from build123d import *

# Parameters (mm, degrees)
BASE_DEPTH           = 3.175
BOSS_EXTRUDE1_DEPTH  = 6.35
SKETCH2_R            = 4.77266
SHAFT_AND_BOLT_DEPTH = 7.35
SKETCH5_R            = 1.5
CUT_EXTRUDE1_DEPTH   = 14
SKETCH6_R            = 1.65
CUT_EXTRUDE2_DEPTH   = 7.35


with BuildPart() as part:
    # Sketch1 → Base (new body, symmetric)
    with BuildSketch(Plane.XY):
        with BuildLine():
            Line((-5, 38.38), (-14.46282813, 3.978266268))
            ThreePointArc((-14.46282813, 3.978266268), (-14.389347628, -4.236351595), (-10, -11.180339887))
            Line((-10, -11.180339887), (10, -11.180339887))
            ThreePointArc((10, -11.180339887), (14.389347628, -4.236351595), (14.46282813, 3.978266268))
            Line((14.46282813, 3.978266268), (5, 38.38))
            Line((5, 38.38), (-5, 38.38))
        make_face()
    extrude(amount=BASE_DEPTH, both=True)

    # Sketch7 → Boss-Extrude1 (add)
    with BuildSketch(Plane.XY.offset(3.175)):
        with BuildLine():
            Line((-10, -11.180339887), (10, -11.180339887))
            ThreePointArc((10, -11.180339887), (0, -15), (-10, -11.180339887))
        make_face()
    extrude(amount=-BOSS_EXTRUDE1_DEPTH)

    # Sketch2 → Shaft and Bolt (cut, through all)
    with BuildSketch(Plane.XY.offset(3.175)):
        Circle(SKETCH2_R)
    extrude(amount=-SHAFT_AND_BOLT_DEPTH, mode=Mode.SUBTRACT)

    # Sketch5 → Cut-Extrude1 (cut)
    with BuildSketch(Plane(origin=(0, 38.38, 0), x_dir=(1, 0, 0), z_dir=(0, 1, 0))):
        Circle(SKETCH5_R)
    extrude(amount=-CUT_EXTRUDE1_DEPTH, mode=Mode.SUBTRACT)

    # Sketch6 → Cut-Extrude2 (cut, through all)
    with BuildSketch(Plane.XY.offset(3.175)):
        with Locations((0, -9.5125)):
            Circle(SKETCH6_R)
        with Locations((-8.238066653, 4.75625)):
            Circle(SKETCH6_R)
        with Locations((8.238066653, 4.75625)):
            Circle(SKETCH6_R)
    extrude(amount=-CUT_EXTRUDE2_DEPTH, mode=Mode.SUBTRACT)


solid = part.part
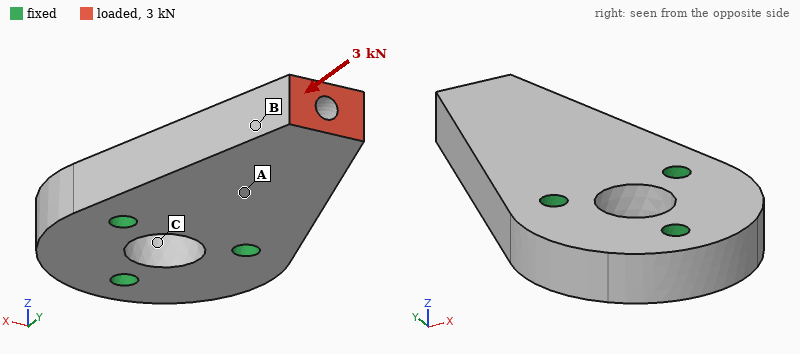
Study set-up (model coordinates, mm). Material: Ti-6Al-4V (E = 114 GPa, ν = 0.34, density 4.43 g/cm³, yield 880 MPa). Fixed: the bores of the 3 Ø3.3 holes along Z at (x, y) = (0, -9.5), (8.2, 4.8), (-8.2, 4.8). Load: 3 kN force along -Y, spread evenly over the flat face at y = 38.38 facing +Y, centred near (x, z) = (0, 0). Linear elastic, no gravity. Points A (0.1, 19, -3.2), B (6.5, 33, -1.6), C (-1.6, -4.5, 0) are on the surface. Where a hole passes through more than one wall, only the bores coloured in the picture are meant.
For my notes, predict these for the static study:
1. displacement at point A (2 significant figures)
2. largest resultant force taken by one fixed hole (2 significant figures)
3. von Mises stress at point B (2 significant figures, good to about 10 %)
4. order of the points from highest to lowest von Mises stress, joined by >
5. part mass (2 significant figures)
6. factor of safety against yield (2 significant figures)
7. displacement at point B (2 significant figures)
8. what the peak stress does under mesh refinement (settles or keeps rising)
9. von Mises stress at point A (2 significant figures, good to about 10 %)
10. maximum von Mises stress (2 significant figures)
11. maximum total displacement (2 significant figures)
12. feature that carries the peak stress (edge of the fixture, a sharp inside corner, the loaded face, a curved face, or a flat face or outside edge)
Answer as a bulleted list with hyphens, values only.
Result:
- 3.1 µm
- 1.5 kN
- 33 MPa
- B > A > C
- 29 g
- 14
- 6.3 µm
- settles
- 22 MPa
- 61 MPa
- 9.6 µm
- a curved face
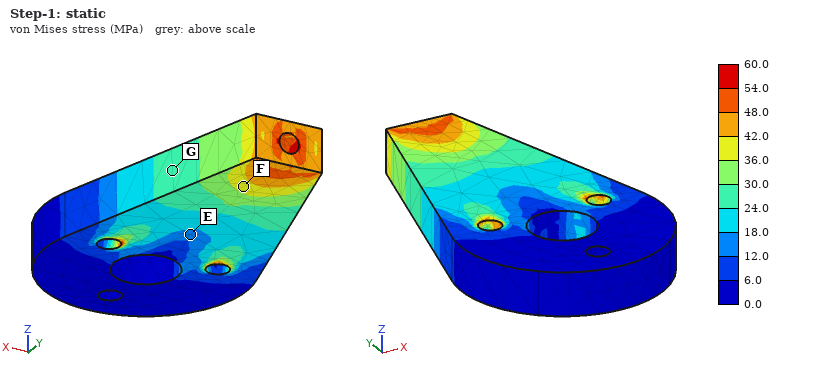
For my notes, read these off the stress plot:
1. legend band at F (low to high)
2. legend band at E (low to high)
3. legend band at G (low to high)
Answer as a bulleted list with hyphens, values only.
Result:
- 36.0 to 42.0 MPa
- 12.0 to 18.0 MPa
- 24.0 to 30.0 MPa
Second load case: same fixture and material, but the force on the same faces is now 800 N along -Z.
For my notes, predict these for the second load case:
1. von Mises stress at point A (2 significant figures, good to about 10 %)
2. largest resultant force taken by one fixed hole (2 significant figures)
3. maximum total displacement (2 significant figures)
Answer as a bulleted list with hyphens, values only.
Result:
- 110 MPa
- 490 N
- 0.21 mm
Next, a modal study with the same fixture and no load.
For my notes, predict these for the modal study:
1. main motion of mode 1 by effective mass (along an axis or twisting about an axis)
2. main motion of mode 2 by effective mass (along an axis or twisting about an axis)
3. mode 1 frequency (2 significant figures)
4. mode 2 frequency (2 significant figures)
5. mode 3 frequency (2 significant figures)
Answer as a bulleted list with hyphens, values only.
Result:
- along Z
- along X
- 5900 Hz
- 18 kHz
- 22 kHz
